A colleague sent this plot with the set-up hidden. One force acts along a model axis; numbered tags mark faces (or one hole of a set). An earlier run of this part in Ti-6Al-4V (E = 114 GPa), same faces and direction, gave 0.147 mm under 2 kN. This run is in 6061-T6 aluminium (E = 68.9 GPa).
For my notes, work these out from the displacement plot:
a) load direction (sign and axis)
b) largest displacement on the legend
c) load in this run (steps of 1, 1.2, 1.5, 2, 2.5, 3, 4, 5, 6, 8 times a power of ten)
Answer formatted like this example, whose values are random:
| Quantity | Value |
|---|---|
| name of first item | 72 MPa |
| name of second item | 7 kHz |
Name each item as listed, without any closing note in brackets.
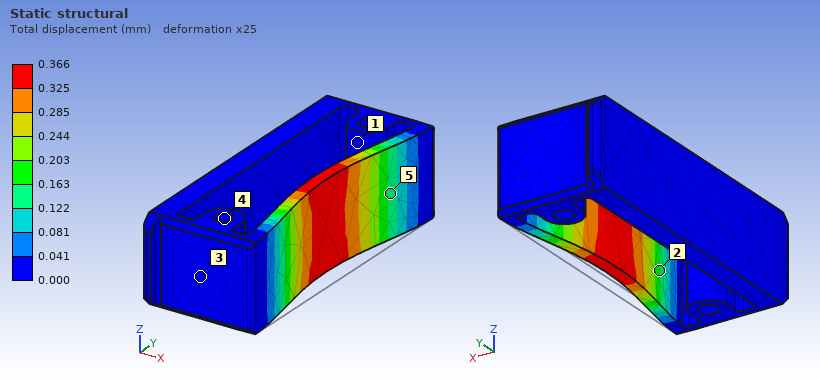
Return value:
| Quantity | Value |
|---|---|
| load direction | -X |
| largest displacement on the legend | 0.366 mm |
| load in this run | 3 kN |
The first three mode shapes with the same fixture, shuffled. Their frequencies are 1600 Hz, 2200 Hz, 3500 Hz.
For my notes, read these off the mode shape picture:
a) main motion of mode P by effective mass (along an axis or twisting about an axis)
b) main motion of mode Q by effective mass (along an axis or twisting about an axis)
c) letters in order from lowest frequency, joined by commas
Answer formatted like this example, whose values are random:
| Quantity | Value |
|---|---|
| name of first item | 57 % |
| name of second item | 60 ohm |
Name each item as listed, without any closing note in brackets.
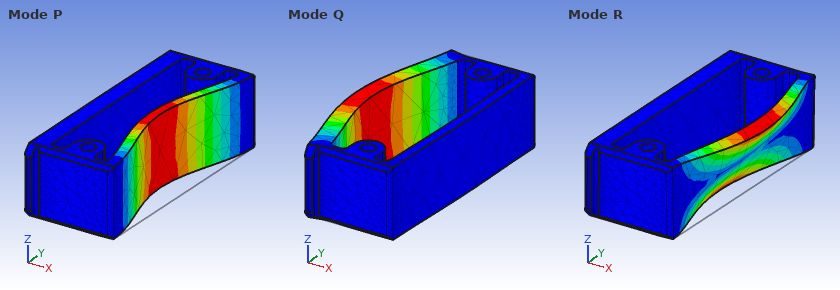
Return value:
| Quantity | Value |
|---|---|
| main motion of mode P by effective mass | along X |
| main motion of mode Q by effective mass | along X |
| letters in order from lowest frequency, joined by commas | P, Q, R |
